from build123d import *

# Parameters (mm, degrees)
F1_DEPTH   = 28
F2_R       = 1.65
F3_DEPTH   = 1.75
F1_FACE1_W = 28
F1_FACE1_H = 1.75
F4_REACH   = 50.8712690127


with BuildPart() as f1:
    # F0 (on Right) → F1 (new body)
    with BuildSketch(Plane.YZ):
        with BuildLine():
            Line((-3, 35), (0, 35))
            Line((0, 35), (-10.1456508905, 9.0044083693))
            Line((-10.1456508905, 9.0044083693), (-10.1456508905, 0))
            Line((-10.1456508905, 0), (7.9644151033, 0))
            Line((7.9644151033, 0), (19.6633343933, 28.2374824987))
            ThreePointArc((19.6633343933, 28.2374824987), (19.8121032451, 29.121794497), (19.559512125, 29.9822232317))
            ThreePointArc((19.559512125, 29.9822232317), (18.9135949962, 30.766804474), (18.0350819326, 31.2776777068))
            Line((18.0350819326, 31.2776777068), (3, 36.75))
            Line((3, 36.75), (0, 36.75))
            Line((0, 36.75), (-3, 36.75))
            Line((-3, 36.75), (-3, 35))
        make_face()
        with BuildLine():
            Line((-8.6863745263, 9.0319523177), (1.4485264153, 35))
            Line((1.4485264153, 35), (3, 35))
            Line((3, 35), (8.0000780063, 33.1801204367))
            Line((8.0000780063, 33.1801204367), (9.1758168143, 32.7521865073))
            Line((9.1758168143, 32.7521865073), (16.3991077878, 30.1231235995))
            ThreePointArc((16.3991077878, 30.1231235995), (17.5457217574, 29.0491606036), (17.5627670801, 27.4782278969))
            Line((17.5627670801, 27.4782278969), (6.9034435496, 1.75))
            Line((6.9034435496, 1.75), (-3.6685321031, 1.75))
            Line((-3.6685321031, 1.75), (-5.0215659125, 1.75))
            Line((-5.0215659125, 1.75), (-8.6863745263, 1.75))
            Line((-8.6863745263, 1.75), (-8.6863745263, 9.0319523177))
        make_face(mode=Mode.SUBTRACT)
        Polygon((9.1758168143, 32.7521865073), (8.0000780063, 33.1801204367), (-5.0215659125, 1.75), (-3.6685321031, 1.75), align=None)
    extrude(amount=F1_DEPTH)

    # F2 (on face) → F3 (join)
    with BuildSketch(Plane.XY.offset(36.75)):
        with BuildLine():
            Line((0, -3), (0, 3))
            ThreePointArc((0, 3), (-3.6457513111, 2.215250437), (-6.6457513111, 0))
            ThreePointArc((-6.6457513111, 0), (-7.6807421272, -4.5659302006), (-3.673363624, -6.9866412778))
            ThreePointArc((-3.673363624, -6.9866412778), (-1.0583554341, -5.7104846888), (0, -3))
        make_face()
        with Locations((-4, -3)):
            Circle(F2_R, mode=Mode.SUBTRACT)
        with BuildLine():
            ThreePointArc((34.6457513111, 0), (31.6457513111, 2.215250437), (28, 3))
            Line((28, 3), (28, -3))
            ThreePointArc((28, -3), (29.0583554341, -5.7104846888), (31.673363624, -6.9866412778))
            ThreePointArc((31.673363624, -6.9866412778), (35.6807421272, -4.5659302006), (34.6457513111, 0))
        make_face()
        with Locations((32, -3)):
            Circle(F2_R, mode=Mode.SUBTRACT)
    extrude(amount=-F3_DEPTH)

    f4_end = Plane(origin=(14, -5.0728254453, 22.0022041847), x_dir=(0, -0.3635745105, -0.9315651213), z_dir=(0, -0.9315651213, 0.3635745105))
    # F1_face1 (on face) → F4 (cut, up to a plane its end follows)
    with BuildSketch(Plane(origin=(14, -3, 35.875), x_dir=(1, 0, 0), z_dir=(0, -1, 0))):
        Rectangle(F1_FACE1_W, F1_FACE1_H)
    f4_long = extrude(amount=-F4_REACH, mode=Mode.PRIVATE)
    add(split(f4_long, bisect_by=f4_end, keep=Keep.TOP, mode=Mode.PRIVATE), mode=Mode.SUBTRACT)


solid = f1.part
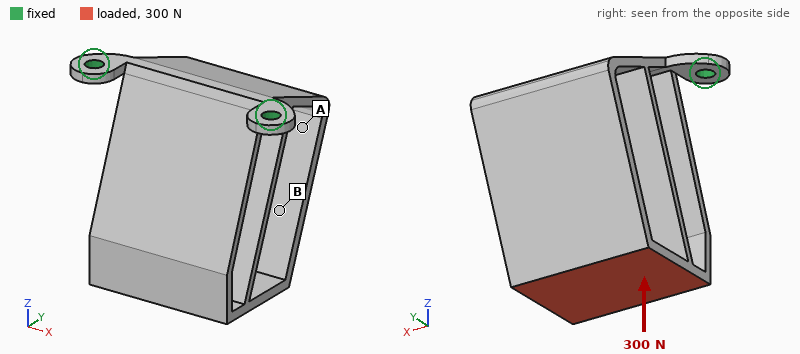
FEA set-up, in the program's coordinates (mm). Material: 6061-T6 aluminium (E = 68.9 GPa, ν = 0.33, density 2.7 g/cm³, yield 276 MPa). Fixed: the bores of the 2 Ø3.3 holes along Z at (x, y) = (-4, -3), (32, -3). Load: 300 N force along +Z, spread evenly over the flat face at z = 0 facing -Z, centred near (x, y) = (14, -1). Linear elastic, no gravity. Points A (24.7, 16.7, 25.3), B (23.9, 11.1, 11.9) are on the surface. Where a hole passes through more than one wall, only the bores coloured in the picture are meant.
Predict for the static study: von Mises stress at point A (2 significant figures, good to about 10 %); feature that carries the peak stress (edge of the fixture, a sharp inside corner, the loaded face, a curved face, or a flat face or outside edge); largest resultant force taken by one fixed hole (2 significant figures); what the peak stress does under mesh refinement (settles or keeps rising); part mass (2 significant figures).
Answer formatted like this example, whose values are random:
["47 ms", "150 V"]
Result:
["33 MPa", "a sharp inside corner", "170 N", "keeps rising", "16 g"]
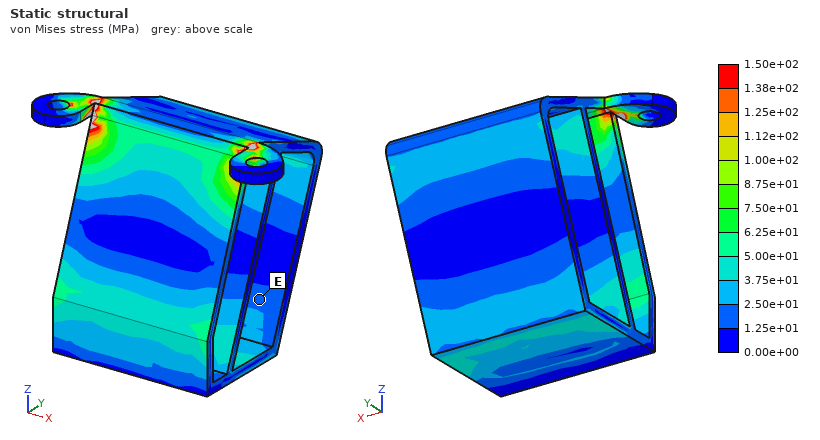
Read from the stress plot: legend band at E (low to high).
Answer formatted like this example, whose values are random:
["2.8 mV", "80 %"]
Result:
["1.25e+01 to 2.50e+01 MPa"]
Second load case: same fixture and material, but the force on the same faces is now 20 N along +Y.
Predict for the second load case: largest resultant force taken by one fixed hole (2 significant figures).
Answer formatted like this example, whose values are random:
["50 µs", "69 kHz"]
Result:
["24 N"]
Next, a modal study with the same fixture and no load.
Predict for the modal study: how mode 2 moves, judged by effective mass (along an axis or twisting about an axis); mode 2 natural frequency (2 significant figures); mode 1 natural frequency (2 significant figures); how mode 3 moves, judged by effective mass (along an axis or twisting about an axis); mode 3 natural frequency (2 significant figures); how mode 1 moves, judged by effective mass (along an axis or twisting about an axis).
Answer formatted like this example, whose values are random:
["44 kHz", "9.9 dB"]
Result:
["along X", "1900 Hz", "330 Hz", "along Z", "2300 Hz", "along Y"]
